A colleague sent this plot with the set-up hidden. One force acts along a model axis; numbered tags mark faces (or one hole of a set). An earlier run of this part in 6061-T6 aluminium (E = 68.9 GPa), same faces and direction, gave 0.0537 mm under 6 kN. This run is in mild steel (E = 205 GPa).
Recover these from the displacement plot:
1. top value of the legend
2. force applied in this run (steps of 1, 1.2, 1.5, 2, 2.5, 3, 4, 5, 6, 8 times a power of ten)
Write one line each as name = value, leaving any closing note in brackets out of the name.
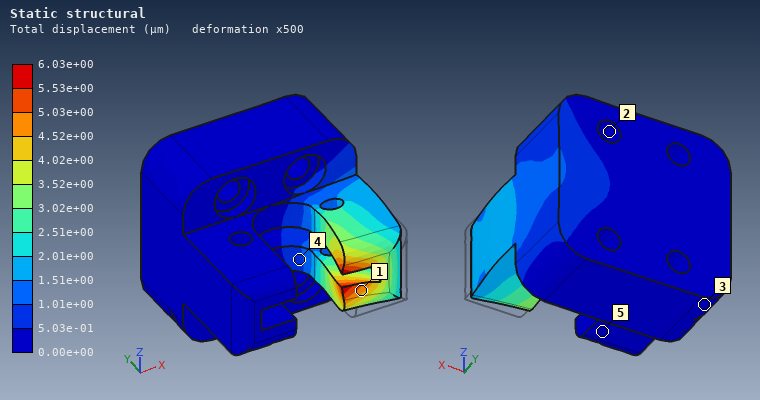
top value of the legend = 6.03e+00 µm
force applied in this run = 2 kN
